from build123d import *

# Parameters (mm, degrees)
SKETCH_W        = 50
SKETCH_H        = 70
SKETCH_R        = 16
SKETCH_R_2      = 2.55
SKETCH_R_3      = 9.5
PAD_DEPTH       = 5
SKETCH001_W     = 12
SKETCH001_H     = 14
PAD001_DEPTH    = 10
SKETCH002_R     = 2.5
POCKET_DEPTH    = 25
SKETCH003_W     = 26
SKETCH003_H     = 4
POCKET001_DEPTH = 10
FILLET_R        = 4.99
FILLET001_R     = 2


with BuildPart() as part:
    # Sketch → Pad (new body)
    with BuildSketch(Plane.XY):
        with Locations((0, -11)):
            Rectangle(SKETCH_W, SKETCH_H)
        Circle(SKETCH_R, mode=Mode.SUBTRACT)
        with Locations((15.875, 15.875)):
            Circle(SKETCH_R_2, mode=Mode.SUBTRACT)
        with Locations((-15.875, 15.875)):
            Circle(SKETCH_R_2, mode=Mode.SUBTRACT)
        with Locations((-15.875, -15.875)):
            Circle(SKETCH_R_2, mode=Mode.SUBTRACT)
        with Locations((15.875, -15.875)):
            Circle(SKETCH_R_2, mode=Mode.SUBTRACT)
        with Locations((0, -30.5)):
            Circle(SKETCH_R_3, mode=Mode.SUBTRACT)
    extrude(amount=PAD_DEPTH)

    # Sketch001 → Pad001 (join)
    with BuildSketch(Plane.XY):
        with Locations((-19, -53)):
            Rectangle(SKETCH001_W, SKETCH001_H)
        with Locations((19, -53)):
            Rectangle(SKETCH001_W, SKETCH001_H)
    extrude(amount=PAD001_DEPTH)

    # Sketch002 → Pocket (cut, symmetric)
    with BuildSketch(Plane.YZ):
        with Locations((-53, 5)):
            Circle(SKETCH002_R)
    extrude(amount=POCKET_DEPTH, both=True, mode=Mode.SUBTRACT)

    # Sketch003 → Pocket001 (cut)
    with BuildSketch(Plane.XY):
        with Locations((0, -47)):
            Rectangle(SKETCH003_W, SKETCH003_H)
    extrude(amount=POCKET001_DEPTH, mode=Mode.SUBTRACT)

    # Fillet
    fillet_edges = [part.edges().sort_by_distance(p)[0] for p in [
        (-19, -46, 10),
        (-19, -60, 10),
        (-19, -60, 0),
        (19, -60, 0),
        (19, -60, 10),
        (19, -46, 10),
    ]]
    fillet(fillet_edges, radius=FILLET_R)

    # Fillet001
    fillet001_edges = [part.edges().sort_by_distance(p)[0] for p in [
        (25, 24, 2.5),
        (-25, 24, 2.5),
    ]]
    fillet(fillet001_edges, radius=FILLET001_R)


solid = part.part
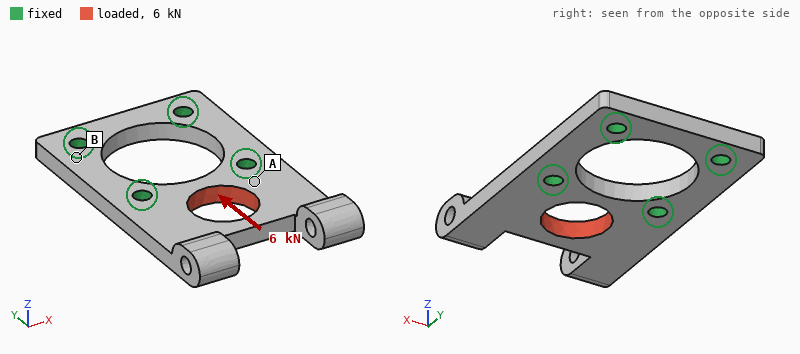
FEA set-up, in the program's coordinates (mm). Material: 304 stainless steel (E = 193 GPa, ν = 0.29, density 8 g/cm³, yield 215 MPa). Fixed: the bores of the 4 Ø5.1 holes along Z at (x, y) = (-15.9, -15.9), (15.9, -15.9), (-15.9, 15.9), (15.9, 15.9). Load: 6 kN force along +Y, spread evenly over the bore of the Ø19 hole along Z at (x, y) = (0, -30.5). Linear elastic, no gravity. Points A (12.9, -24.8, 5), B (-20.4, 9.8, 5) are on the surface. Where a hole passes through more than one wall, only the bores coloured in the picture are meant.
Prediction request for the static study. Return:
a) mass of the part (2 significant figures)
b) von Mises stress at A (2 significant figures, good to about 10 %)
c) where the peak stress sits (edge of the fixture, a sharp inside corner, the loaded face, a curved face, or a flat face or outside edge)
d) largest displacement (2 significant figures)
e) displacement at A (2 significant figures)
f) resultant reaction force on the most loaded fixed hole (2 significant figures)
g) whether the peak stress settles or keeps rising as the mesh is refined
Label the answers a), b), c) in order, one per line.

a) 110 g
b) 56 MPa
c) edge of the fixture
d) 9.5 µm
e) 2.1 µm
f) 3.1 kN
g) keeps rising
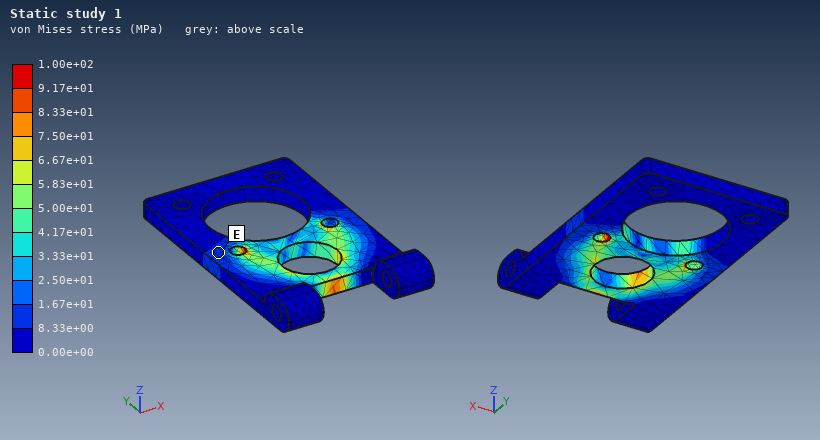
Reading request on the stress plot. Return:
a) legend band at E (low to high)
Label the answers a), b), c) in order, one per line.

a) 8.33e+00 to 1.67e+01 MPa
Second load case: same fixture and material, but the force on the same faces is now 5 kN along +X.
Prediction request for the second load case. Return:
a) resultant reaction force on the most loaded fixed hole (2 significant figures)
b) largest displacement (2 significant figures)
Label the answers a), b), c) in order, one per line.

a) 2.8 kN
b) 31 µm
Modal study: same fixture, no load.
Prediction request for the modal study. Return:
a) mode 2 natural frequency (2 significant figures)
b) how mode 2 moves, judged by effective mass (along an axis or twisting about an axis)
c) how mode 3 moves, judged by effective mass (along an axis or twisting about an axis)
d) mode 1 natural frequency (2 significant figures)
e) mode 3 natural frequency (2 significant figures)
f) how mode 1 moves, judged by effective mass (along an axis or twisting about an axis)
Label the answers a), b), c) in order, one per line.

a) 2800 Hz
b) twisting about Y
c) along X
d) 2000 Hz
e) 6900 Hz
f) along Z
